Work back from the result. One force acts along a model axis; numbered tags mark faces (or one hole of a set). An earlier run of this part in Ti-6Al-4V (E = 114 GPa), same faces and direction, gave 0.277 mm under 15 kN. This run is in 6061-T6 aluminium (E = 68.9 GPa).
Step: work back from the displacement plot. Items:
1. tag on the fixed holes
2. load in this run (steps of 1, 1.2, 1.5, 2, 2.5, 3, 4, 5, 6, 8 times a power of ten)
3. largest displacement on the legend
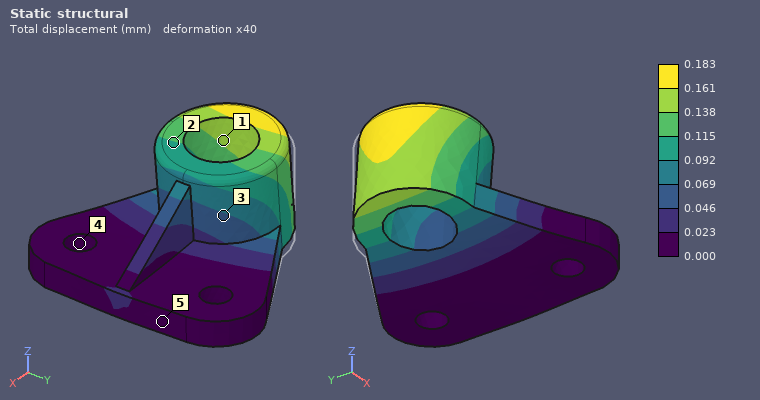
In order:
4
6 kN
0.183 mm
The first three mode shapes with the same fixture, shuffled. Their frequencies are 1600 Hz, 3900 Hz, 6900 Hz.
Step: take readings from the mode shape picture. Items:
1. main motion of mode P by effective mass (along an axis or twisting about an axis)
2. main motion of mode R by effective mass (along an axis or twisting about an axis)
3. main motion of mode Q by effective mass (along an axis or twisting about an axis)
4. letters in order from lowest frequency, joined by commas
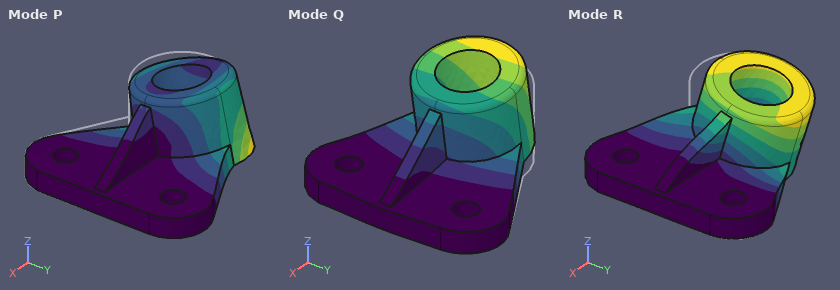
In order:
along Y
along Y
along Z
Q, R, P
